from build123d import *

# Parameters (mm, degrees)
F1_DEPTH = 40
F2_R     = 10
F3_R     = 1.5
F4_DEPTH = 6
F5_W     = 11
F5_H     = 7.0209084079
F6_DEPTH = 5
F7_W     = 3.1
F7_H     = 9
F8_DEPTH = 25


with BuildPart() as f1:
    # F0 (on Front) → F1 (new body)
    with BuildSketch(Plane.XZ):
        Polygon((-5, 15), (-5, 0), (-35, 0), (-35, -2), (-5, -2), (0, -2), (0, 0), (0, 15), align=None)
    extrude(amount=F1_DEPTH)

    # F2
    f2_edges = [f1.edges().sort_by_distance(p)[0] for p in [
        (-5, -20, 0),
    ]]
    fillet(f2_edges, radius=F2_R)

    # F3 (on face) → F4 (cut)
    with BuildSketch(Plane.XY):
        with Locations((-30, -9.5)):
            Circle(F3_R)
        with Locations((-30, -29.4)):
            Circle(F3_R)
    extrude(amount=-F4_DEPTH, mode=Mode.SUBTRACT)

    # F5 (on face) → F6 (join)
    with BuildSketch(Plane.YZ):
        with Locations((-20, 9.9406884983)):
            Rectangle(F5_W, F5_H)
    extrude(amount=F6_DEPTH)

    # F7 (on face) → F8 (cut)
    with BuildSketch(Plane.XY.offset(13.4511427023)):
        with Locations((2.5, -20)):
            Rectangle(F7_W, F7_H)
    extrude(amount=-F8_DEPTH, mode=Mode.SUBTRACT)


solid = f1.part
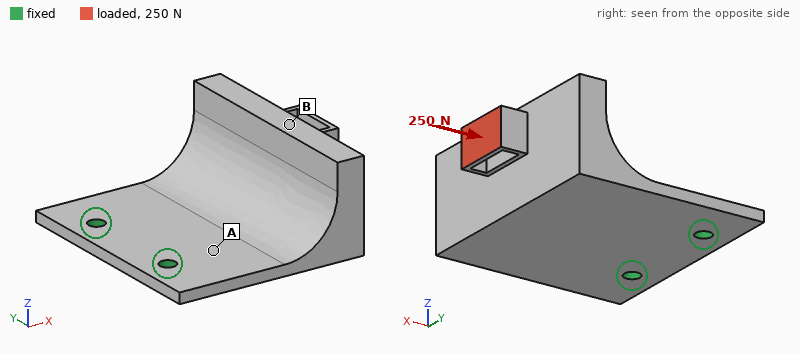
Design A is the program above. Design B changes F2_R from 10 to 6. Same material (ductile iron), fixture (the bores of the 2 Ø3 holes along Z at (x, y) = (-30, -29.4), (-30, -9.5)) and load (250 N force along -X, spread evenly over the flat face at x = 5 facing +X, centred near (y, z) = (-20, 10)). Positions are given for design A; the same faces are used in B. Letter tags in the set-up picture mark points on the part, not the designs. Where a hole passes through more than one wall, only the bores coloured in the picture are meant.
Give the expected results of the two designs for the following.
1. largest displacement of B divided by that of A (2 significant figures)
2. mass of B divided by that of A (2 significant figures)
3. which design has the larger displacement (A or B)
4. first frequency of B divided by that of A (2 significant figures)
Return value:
1.1
0.92
B
1.0
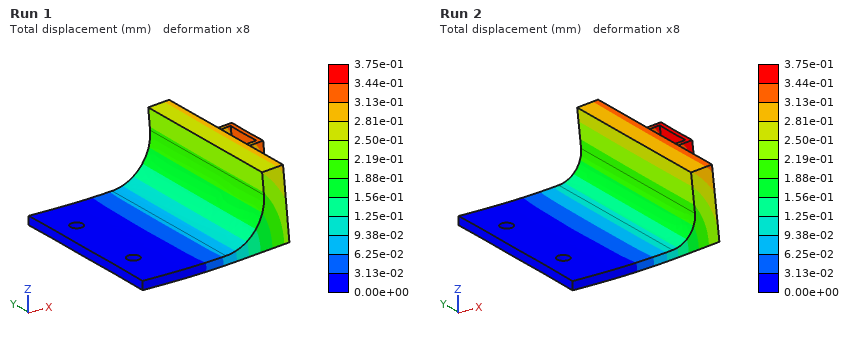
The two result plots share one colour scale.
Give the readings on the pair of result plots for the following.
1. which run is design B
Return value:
Run 2
